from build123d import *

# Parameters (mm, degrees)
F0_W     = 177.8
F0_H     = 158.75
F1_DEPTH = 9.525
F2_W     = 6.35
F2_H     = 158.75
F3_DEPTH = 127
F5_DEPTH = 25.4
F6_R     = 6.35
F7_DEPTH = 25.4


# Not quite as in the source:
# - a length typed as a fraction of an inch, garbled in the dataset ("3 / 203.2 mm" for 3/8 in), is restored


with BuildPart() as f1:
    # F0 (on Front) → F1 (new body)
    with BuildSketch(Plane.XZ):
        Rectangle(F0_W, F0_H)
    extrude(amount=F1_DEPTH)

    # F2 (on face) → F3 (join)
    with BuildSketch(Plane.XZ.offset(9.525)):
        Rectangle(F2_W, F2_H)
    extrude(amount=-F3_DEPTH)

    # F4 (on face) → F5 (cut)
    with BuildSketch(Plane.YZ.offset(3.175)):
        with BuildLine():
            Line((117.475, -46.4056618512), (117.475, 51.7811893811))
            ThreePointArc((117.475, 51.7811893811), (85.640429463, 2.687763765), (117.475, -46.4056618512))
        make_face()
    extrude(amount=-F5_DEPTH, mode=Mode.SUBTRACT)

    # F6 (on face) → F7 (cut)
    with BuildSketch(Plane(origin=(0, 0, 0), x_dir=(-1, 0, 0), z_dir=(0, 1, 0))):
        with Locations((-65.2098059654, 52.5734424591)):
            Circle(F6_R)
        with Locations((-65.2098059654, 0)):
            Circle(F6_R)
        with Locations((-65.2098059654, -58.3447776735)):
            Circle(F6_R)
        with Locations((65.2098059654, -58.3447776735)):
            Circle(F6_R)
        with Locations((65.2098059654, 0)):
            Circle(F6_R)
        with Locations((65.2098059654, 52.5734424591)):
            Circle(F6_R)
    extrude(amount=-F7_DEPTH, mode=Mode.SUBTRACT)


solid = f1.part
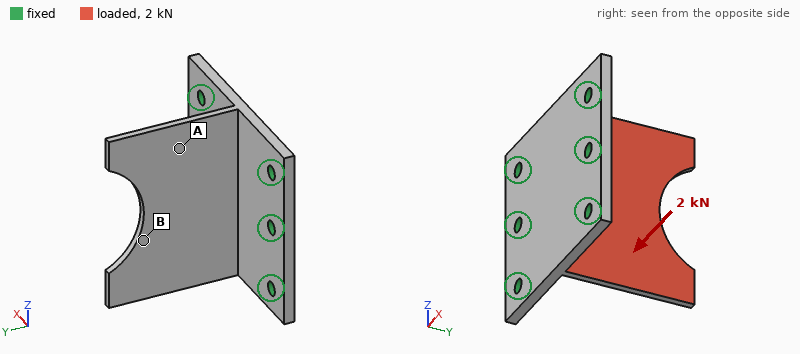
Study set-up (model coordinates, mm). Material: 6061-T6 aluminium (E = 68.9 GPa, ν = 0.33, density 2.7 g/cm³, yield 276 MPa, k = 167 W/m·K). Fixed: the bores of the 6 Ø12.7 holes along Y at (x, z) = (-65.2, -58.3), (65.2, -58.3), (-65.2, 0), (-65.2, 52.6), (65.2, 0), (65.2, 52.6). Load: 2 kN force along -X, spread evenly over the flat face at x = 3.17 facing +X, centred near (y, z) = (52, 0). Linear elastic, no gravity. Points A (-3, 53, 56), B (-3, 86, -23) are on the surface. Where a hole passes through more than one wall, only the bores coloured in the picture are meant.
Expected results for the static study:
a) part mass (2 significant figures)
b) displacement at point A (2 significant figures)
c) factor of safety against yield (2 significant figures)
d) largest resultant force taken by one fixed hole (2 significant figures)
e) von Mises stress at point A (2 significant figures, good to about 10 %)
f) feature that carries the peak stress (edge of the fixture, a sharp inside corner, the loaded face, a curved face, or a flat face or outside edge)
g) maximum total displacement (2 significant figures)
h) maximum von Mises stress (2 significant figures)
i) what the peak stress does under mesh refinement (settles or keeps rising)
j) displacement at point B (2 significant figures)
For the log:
990 g
0.51 mm
3.4
590 N
23 MPa
the loaded face
1.6 mm
82 MPa
settles
1.0 mm
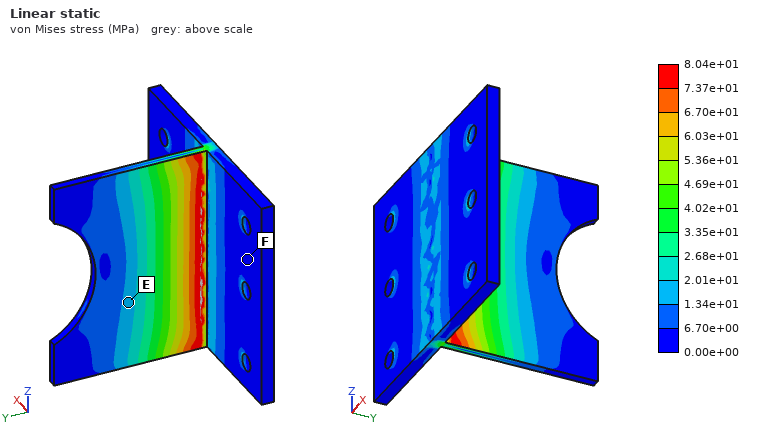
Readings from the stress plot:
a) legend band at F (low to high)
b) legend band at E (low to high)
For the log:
0.00e+00 to 6.70e+00 MPa
1.34e+01 to 2.01e+01 MPa
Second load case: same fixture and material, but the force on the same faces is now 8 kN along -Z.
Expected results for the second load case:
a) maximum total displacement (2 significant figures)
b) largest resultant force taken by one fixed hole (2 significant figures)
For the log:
0.44 mm
2.5 kN
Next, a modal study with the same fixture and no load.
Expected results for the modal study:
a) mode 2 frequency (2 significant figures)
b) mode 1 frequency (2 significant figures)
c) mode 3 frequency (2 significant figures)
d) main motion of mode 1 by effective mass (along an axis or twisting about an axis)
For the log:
680 Hz
450 Hz
1400 Hz
along X
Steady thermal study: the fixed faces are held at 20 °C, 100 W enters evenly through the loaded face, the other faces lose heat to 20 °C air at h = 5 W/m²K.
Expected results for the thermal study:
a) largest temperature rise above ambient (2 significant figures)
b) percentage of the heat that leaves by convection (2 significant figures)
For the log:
46 K
4.7 %
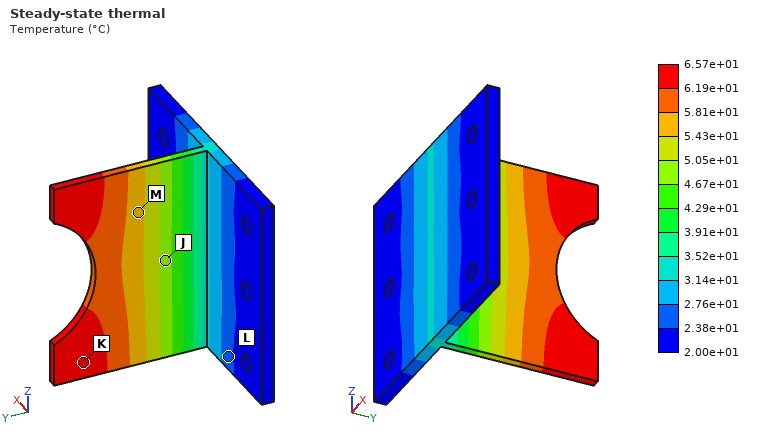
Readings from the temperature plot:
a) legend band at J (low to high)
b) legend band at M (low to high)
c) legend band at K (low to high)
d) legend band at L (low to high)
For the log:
4.67e+01 to 5.05e+01 °C
5.43e+01 to 5.81e+01 °C
6.19e+01 to 6.57e+01 °C
2.38e+01 to 2.76e+01 °C
